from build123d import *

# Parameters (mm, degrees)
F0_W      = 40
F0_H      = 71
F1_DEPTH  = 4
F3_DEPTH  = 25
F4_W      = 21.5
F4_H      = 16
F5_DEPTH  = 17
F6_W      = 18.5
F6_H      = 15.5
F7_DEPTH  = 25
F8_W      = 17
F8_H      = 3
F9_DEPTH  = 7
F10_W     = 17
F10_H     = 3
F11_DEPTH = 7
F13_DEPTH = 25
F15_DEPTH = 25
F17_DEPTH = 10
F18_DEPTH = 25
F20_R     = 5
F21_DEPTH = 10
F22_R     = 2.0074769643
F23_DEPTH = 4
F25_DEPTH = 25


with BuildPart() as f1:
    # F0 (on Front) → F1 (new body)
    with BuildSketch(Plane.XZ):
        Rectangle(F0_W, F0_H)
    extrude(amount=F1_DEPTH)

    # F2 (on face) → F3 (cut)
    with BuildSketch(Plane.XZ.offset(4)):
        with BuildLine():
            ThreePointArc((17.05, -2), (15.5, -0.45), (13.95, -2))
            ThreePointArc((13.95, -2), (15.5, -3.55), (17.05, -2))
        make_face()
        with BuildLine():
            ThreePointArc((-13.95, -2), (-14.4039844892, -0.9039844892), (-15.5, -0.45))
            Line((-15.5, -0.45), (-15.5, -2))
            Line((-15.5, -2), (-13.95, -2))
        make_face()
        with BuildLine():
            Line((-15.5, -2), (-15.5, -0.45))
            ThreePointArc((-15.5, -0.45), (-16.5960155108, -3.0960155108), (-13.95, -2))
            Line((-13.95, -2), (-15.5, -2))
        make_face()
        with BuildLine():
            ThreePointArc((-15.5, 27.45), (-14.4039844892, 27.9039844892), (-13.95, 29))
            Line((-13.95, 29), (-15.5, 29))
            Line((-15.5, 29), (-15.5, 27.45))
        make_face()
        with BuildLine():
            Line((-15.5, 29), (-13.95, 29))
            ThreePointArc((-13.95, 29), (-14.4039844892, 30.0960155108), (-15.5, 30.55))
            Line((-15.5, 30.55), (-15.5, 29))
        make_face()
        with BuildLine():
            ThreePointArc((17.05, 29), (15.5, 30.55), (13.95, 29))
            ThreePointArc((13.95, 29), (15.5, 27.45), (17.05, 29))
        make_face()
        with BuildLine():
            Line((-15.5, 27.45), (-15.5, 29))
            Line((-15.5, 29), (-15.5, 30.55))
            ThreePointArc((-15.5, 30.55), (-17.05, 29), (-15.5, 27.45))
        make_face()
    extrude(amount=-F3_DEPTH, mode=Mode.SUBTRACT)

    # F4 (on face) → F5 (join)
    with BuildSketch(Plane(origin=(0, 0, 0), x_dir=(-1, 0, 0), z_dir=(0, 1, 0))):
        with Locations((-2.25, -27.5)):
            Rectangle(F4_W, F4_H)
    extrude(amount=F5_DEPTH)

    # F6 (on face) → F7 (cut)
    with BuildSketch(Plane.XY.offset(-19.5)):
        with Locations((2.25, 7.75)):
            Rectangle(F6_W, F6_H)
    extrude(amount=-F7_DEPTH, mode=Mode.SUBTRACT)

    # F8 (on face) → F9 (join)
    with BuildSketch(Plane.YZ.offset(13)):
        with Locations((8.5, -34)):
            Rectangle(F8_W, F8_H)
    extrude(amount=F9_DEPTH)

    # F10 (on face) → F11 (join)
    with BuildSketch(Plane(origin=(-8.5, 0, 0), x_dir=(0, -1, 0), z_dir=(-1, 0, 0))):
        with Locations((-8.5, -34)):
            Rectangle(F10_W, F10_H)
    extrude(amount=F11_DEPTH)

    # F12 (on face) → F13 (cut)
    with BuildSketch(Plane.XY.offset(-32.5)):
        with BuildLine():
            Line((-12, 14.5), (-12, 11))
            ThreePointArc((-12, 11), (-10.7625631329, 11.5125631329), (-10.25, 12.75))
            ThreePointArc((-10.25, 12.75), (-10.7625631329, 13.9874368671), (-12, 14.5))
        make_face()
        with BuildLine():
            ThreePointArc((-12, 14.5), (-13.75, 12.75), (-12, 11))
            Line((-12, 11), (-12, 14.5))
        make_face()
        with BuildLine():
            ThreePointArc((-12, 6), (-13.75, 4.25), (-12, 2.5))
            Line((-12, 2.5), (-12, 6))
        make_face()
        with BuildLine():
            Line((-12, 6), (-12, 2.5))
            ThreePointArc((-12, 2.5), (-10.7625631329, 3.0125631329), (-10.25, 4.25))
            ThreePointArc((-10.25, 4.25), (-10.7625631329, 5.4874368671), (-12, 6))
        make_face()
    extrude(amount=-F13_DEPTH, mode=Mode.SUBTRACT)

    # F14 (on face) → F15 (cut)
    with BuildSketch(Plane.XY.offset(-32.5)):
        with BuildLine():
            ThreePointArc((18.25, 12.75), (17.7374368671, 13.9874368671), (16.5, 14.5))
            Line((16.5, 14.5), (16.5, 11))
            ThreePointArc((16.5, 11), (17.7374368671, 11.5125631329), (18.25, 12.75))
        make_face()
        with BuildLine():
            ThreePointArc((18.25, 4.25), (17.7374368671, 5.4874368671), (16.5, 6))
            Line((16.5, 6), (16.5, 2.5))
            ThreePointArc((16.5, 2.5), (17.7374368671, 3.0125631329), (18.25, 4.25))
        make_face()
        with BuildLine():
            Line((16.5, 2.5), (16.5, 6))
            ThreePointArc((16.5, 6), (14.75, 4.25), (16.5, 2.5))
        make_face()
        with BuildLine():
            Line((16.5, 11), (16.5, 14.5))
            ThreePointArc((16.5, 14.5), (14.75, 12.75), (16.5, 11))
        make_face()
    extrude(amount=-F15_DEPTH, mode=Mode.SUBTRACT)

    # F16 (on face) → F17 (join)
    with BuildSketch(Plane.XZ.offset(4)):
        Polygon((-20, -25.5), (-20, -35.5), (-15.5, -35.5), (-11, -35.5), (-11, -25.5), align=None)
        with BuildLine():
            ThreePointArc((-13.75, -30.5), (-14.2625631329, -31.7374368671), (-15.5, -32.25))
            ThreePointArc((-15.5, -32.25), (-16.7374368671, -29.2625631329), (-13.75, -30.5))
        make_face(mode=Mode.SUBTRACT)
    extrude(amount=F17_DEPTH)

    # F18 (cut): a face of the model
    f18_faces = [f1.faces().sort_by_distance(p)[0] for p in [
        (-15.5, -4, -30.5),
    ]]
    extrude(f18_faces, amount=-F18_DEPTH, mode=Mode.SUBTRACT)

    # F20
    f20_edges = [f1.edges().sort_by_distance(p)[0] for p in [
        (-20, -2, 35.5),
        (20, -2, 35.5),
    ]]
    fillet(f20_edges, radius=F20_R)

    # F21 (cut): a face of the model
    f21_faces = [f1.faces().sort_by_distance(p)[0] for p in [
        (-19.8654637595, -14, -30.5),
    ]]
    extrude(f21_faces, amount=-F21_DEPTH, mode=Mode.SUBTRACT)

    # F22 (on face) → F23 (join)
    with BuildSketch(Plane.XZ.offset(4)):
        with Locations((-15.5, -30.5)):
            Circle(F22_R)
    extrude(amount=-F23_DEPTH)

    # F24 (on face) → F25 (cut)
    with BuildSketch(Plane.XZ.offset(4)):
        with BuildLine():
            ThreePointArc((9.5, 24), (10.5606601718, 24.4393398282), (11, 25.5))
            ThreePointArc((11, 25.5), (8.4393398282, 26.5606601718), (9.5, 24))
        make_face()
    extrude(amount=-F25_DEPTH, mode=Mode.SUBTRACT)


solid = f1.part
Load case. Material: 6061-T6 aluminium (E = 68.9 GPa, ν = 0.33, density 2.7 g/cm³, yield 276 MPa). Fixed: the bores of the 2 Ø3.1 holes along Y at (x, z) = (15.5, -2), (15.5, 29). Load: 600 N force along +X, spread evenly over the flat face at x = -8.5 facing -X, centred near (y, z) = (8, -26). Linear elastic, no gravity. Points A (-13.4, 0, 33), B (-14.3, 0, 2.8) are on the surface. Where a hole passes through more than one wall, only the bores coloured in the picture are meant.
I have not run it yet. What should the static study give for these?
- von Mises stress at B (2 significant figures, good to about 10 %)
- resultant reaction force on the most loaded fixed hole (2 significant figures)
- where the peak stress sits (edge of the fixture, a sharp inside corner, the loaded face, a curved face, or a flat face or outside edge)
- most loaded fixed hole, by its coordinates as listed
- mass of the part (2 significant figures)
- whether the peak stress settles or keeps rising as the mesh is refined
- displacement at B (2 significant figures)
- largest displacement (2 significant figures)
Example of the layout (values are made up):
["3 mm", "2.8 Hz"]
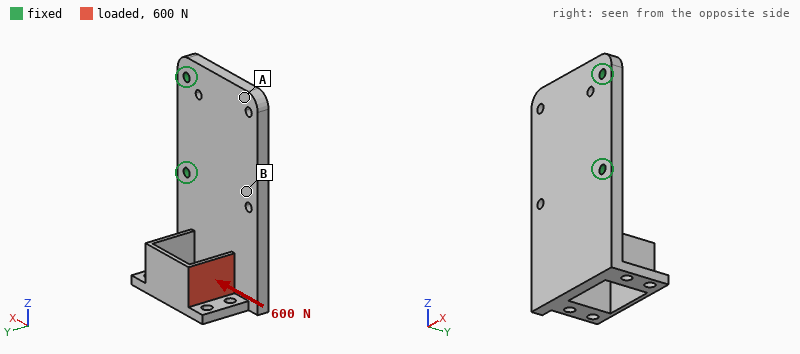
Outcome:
["26 MPa", "1.0 kN", "edge of the fixture", "(15.5, -2)", "35 g", "keeps rising", "0.14 mm", "0.43 mm"]
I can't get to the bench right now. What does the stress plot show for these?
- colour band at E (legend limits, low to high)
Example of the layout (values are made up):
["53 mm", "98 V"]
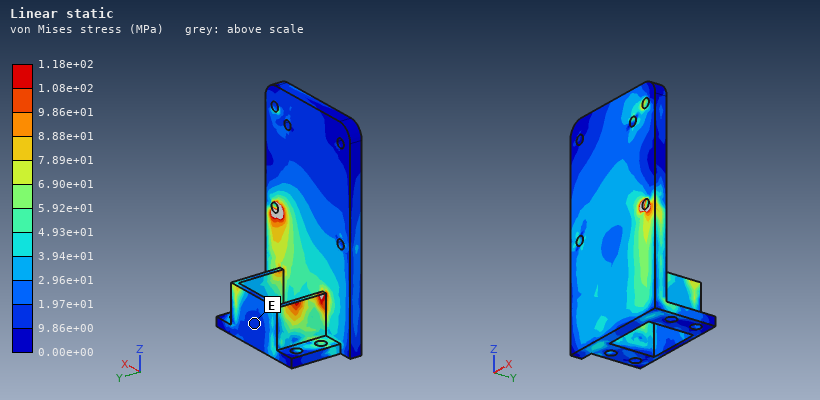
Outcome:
["9.86e+00 to 1.97e+01 MPa"]
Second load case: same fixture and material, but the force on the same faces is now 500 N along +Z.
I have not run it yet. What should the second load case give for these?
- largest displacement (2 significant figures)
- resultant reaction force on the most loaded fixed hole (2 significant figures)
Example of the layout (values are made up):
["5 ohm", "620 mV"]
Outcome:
["0.38 mm", "450 N"]
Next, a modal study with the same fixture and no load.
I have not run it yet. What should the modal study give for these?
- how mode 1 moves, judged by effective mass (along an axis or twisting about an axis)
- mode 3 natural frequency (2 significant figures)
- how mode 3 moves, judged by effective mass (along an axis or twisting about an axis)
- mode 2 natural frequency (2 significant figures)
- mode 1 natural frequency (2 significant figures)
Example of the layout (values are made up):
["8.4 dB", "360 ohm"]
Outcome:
["along Y", "3400 Hz", "along Y", "2000 Hz", "1300 Hz"]
